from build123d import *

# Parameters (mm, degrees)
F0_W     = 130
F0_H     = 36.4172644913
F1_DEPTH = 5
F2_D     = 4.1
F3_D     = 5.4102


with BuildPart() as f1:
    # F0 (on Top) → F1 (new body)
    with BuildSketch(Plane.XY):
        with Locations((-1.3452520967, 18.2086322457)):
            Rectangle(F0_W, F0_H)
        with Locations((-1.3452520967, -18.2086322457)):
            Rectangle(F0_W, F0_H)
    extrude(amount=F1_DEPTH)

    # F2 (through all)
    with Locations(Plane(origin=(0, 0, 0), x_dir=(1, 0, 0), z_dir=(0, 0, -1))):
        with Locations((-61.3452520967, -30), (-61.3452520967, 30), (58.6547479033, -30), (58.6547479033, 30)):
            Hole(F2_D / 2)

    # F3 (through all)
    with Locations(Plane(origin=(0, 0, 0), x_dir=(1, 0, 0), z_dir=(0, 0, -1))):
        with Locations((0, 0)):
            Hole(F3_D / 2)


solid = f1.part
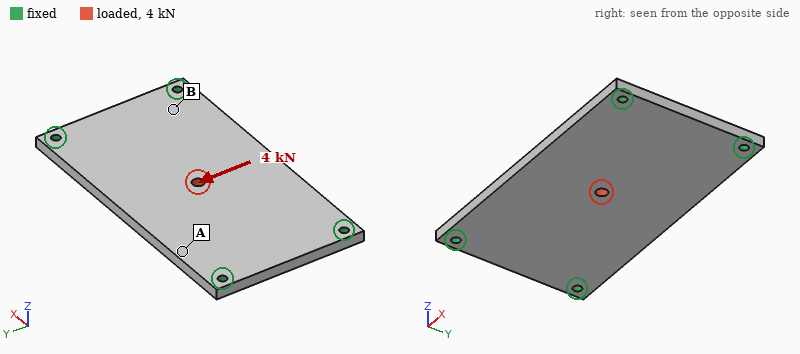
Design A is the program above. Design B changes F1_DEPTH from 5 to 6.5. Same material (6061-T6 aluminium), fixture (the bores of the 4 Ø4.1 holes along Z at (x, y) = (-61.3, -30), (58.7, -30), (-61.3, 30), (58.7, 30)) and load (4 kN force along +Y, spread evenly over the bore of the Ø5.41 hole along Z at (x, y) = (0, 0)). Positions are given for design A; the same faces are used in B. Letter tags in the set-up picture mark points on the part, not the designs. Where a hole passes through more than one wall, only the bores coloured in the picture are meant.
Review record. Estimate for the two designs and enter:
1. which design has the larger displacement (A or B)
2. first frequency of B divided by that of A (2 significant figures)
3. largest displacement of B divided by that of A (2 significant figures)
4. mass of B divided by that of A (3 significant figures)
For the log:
A
1.3
0.77
1.30
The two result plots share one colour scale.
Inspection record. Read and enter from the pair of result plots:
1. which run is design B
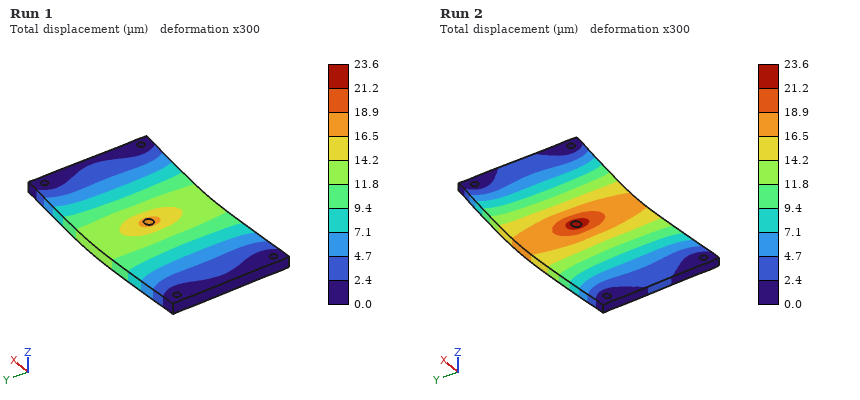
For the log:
Run 1
